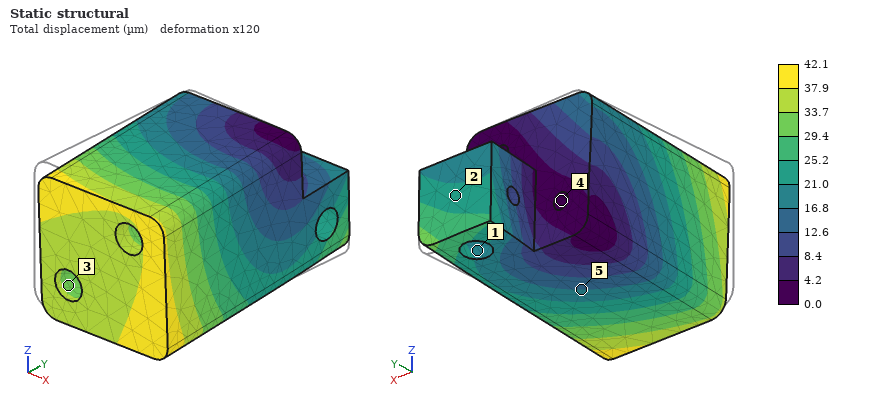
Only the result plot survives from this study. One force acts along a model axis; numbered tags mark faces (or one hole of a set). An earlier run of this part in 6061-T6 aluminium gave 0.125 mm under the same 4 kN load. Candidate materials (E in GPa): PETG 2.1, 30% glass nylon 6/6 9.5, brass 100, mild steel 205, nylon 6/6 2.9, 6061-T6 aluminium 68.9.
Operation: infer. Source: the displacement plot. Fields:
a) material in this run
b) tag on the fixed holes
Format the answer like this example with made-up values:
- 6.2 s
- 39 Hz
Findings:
- mild steel
- 4
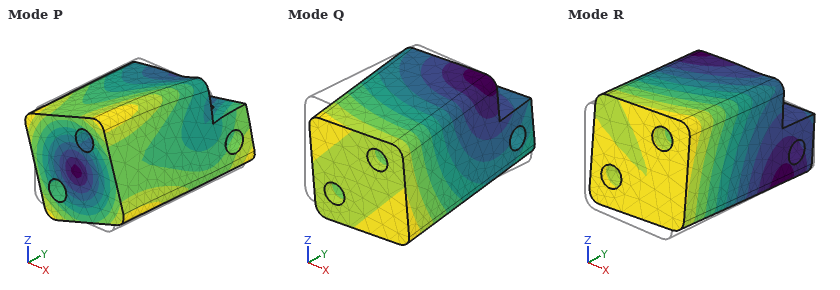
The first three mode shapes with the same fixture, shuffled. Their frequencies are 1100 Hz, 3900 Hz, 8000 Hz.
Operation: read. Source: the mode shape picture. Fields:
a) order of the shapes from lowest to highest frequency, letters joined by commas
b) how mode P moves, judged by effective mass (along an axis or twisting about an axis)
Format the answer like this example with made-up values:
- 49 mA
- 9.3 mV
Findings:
- Q, R, P
- twisting about Y
